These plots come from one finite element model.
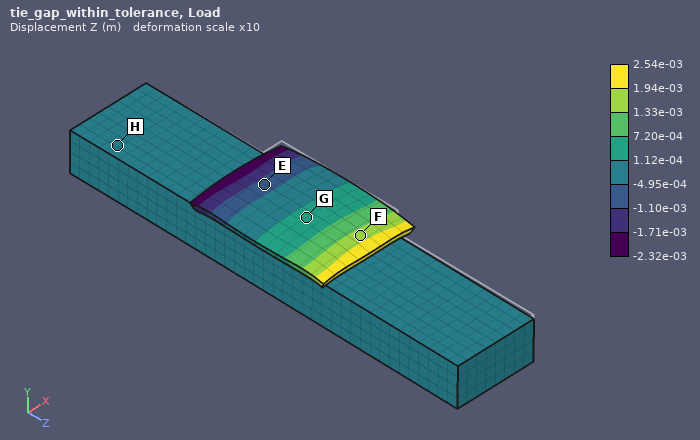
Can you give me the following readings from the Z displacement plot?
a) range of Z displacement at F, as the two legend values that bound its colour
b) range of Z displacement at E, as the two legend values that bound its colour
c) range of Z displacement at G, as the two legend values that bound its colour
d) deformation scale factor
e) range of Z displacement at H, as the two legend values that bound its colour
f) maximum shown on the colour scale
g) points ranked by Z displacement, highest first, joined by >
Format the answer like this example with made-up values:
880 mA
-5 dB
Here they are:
1.33e-03 to 1.94e-03 m
-1.10e-03 to -4.95e-04 m
1.12e-04 to 7.20e-04 m
10
-4.95e-04 to 1.12e-04 m
2.54e-03 m
F > G > H > E
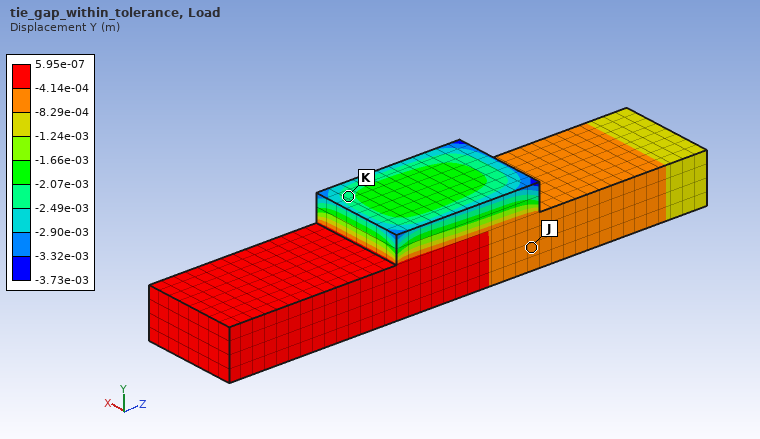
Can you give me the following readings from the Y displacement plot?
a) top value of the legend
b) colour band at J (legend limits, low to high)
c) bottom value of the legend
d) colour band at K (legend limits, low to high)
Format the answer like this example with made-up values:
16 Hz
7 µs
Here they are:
5.95e-07 m
-8.29e-04 to -4.14e-04 m
-3.73e-03 m
-2.49e-03 to -2.07e-03 m
